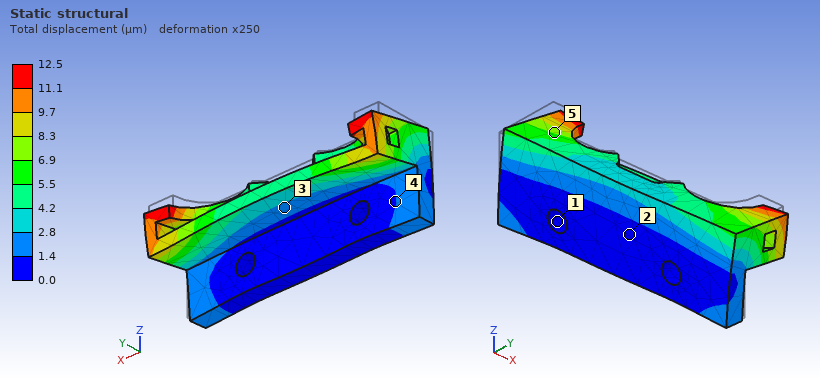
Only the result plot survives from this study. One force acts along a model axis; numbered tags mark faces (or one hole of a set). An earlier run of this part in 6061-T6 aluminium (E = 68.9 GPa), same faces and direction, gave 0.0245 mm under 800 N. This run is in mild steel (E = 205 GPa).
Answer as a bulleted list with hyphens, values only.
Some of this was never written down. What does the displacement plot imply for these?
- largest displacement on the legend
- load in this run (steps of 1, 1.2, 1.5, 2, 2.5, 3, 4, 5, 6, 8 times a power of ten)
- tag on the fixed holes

- 12.5 µm
- 1.2 kN
- 1
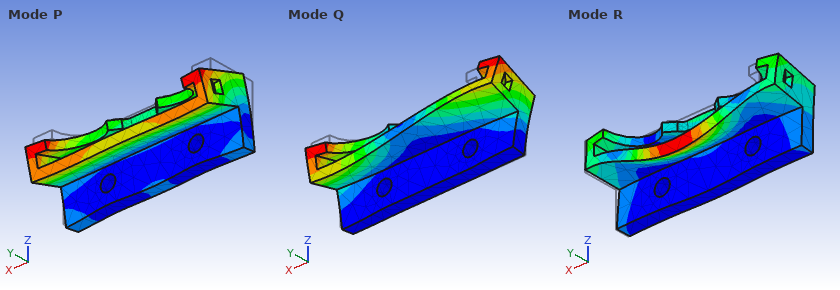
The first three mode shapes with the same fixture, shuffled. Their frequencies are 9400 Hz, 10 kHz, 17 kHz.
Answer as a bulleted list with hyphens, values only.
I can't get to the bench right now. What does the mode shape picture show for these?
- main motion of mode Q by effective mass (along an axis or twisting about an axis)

- twisting about Z
